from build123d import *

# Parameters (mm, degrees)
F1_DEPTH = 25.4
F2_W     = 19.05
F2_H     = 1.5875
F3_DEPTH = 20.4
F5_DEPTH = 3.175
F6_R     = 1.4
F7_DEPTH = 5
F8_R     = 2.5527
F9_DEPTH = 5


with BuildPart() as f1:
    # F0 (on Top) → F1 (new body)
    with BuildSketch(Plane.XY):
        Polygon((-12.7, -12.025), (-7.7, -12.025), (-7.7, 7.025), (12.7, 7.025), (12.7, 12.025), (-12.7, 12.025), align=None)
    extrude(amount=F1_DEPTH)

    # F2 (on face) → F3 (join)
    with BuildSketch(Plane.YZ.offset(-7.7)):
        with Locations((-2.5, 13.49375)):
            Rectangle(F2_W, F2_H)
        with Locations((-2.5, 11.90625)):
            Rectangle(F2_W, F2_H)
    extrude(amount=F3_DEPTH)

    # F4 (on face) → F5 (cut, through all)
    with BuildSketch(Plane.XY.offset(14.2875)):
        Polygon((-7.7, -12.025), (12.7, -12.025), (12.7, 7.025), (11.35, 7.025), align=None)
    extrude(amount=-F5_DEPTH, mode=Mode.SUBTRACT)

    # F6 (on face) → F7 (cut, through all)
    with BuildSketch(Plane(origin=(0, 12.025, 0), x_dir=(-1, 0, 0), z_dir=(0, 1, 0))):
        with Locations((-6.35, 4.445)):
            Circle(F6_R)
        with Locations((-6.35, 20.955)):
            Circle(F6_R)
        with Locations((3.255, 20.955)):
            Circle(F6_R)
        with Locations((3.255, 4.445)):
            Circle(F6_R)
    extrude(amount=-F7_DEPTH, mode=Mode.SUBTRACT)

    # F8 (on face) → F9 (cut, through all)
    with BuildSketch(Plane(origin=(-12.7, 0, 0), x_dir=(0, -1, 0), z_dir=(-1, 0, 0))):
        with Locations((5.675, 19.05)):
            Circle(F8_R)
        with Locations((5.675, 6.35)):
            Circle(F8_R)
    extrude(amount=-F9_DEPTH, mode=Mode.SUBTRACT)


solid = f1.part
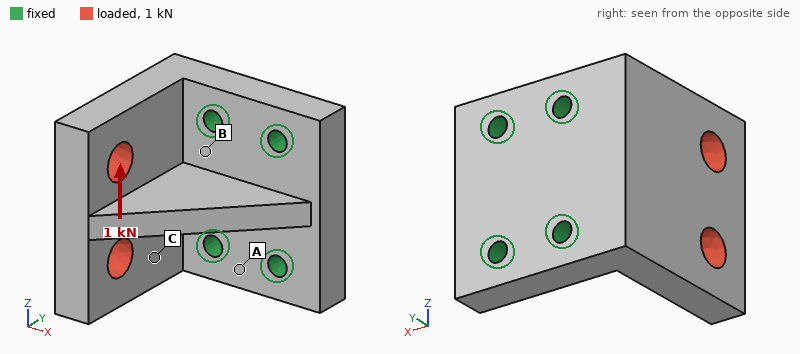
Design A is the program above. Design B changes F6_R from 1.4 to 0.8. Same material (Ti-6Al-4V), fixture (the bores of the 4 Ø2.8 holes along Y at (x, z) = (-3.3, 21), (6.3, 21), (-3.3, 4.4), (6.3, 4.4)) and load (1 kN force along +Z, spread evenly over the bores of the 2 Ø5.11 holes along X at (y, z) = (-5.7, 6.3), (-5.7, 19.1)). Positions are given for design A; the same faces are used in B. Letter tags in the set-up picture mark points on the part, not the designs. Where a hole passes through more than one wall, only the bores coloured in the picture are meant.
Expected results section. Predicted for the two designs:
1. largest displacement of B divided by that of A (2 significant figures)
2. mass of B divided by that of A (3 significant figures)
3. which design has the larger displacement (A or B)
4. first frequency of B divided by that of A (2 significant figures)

1.2
1.01
B
0.91
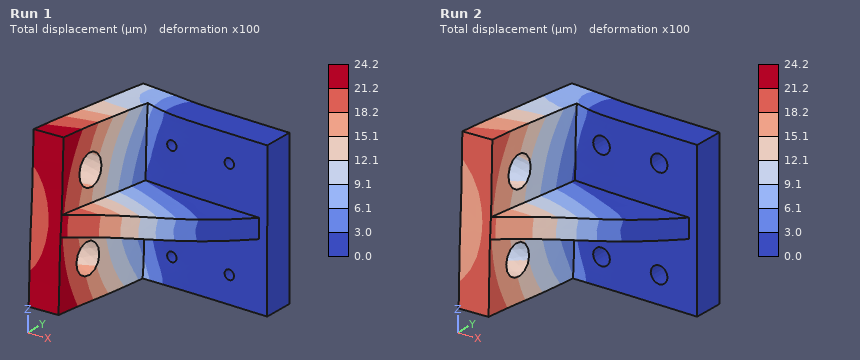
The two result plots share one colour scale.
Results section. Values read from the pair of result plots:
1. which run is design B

Run 1
